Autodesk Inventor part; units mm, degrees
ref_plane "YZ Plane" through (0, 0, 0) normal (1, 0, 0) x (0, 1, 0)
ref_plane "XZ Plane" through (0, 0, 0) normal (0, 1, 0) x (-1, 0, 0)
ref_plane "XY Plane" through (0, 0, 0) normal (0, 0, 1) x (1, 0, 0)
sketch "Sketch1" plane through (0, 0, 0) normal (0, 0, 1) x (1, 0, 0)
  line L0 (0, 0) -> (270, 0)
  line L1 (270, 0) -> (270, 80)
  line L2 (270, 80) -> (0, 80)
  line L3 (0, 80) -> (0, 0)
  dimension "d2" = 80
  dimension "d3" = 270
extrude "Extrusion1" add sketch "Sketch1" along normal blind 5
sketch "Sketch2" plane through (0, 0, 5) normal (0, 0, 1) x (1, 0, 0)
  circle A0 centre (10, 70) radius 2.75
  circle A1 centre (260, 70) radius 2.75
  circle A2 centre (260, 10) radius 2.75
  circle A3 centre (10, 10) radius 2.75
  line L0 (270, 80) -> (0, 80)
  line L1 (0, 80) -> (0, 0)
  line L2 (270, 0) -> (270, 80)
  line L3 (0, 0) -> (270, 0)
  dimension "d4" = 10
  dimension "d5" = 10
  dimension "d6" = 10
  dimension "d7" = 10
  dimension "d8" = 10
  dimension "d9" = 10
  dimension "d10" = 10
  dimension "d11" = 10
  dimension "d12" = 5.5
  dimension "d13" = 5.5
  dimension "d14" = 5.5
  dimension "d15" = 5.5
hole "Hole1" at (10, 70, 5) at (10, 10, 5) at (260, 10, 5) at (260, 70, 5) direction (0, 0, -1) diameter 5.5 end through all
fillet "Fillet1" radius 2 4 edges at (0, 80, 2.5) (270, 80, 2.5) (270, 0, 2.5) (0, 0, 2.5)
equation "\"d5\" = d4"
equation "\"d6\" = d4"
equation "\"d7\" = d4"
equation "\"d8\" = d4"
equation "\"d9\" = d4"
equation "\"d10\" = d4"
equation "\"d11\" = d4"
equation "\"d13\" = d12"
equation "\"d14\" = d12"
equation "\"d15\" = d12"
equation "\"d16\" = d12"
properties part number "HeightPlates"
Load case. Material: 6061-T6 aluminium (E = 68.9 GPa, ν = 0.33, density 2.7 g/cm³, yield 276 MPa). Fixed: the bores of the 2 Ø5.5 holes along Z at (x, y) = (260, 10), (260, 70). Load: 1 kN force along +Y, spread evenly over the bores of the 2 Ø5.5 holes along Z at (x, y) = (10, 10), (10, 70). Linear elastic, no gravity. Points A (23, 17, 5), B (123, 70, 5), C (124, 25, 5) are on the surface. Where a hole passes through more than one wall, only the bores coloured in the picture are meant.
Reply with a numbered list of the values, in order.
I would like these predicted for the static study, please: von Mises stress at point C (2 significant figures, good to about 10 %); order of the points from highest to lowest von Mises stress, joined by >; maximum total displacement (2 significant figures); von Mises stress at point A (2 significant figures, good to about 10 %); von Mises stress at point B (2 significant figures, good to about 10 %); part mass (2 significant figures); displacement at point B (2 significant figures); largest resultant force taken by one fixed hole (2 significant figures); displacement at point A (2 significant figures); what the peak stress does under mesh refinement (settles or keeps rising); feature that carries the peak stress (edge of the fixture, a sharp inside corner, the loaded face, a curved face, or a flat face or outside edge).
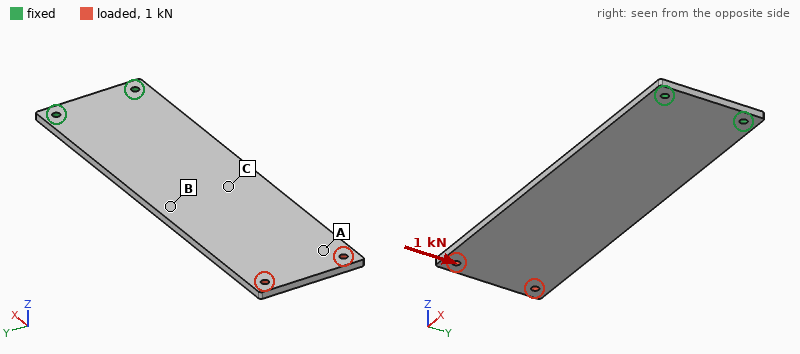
1. 9.8 MPa
2. B > C > A
3. 0.43 mm
4. 5.1 MPa
5. 16 MPa
6. 290 g
7. 0.17 mm
8. 4.1 kN
9. 0.37 mm
10. keeps rising
11. edge of the fixture
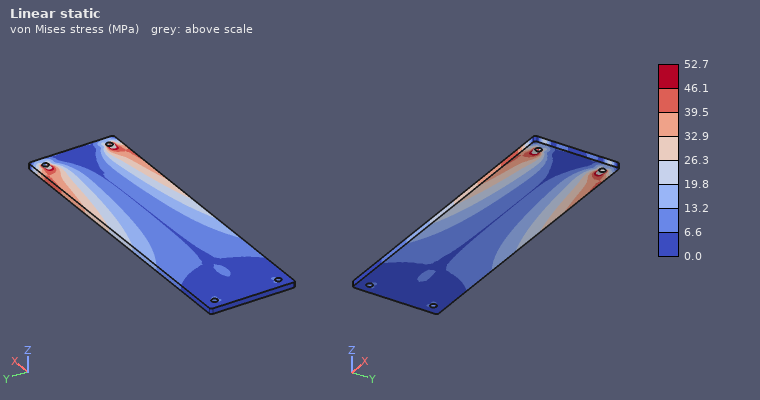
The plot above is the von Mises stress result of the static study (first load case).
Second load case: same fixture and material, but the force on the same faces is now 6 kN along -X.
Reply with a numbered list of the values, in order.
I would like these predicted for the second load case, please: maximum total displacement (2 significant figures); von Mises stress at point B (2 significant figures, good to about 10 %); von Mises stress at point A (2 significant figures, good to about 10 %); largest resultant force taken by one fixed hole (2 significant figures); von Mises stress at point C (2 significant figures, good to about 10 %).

1. 67 µm
2. 15 MPa
3. 21 MPa
4. 3.1 kN
5. 15 MPa
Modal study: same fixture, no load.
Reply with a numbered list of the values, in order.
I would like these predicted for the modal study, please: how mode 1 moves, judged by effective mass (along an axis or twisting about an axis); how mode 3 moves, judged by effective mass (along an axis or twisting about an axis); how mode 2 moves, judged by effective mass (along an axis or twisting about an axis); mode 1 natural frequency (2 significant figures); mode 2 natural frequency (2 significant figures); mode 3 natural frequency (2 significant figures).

1. along Z
2. twisting about X
3. along Z
4. 59 Hz
5. 370 Hz
6. 400 Hz
